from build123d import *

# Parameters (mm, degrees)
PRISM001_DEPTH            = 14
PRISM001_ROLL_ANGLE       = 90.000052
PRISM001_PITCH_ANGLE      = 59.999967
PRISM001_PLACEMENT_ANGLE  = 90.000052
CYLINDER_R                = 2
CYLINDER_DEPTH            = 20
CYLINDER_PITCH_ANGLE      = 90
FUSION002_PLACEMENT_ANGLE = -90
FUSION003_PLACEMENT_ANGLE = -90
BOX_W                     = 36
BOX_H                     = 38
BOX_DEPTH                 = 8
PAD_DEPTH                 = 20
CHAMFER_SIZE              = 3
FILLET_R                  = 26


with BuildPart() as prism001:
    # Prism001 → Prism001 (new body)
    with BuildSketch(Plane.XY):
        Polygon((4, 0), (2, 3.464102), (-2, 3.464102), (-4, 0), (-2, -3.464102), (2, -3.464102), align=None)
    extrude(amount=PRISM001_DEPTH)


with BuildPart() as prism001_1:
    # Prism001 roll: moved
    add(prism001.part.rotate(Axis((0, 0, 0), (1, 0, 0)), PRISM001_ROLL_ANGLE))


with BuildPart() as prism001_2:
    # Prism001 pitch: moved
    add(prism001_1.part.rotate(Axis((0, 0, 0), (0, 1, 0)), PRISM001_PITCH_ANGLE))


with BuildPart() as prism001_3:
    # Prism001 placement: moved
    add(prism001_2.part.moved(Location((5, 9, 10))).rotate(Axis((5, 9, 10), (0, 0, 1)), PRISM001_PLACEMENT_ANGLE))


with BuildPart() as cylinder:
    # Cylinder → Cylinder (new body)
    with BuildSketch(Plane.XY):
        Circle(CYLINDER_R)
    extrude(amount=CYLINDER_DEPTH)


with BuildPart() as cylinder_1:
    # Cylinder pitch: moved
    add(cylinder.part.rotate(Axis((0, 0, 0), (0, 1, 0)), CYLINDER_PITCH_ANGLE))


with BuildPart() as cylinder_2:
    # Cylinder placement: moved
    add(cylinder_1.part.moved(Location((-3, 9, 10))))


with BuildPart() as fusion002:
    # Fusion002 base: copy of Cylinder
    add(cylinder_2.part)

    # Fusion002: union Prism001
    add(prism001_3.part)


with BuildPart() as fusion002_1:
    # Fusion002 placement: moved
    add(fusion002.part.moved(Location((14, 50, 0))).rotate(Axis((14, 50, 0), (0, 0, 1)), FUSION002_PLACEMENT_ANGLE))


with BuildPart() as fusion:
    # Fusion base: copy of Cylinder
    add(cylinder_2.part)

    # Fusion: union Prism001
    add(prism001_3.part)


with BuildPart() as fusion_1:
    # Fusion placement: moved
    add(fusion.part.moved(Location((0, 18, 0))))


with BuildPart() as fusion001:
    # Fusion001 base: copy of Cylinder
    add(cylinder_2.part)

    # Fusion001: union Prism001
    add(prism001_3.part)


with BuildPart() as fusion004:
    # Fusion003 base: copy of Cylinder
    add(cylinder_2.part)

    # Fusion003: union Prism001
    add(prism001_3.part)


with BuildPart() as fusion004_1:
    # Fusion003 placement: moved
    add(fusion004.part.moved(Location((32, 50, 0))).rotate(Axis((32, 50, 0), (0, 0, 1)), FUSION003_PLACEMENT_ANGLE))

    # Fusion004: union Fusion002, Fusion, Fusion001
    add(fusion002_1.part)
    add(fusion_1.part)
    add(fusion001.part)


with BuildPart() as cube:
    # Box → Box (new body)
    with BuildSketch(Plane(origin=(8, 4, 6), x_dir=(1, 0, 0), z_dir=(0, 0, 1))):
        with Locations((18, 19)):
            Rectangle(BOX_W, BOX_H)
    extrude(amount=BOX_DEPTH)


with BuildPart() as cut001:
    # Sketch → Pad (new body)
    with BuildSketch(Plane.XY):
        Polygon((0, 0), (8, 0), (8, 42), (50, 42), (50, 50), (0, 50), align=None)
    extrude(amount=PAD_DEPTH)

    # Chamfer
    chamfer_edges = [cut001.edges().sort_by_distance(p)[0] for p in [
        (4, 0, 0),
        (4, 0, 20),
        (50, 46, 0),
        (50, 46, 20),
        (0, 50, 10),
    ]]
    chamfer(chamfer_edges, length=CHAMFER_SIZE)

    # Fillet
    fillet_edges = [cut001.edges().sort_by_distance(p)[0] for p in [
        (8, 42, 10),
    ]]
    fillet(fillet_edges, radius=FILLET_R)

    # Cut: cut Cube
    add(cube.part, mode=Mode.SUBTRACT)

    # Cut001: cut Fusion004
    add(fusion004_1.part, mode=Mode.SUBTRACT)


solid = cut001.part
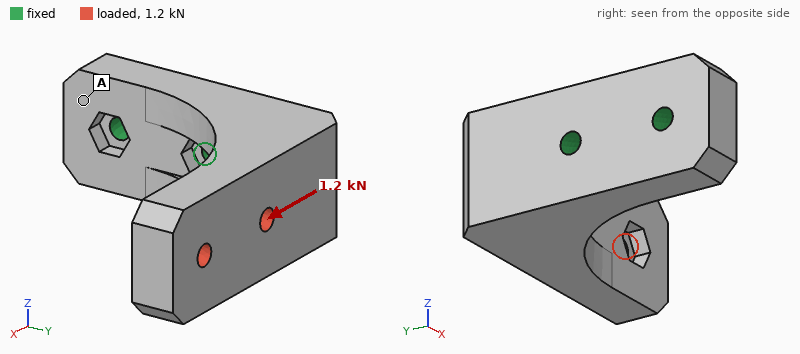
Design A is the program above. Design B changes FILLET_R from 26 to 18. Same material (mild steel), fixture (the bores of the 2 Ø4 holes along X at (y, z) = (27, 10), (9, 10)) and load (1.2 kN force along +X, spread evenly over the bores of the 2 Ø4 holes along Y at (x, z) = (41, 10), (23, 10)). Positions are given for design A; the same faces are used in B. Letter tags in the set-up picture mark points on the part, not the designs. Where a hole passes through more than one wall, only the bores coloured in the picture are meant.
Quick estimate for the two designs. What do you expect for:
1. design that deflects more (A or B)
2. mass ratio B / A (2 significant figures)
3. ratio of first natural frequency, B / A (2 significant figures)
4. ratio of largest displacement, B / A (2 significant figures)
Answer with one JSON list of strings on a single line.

["B", "0.94", "0.86", "1.4"]
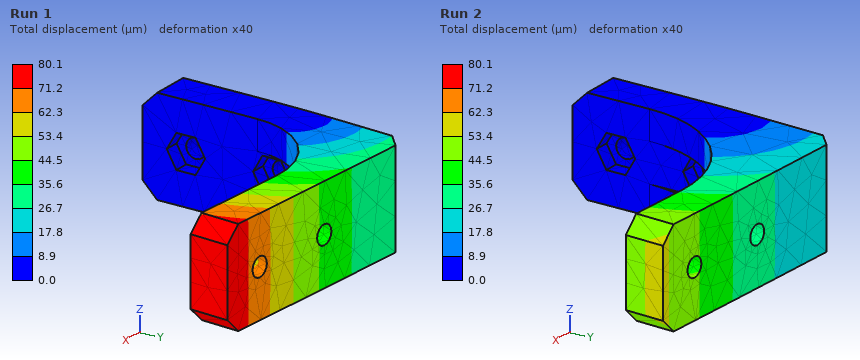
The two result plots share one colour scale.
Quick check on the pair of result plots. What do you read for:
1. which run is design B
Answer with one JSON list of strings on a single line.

["Run 1"]
